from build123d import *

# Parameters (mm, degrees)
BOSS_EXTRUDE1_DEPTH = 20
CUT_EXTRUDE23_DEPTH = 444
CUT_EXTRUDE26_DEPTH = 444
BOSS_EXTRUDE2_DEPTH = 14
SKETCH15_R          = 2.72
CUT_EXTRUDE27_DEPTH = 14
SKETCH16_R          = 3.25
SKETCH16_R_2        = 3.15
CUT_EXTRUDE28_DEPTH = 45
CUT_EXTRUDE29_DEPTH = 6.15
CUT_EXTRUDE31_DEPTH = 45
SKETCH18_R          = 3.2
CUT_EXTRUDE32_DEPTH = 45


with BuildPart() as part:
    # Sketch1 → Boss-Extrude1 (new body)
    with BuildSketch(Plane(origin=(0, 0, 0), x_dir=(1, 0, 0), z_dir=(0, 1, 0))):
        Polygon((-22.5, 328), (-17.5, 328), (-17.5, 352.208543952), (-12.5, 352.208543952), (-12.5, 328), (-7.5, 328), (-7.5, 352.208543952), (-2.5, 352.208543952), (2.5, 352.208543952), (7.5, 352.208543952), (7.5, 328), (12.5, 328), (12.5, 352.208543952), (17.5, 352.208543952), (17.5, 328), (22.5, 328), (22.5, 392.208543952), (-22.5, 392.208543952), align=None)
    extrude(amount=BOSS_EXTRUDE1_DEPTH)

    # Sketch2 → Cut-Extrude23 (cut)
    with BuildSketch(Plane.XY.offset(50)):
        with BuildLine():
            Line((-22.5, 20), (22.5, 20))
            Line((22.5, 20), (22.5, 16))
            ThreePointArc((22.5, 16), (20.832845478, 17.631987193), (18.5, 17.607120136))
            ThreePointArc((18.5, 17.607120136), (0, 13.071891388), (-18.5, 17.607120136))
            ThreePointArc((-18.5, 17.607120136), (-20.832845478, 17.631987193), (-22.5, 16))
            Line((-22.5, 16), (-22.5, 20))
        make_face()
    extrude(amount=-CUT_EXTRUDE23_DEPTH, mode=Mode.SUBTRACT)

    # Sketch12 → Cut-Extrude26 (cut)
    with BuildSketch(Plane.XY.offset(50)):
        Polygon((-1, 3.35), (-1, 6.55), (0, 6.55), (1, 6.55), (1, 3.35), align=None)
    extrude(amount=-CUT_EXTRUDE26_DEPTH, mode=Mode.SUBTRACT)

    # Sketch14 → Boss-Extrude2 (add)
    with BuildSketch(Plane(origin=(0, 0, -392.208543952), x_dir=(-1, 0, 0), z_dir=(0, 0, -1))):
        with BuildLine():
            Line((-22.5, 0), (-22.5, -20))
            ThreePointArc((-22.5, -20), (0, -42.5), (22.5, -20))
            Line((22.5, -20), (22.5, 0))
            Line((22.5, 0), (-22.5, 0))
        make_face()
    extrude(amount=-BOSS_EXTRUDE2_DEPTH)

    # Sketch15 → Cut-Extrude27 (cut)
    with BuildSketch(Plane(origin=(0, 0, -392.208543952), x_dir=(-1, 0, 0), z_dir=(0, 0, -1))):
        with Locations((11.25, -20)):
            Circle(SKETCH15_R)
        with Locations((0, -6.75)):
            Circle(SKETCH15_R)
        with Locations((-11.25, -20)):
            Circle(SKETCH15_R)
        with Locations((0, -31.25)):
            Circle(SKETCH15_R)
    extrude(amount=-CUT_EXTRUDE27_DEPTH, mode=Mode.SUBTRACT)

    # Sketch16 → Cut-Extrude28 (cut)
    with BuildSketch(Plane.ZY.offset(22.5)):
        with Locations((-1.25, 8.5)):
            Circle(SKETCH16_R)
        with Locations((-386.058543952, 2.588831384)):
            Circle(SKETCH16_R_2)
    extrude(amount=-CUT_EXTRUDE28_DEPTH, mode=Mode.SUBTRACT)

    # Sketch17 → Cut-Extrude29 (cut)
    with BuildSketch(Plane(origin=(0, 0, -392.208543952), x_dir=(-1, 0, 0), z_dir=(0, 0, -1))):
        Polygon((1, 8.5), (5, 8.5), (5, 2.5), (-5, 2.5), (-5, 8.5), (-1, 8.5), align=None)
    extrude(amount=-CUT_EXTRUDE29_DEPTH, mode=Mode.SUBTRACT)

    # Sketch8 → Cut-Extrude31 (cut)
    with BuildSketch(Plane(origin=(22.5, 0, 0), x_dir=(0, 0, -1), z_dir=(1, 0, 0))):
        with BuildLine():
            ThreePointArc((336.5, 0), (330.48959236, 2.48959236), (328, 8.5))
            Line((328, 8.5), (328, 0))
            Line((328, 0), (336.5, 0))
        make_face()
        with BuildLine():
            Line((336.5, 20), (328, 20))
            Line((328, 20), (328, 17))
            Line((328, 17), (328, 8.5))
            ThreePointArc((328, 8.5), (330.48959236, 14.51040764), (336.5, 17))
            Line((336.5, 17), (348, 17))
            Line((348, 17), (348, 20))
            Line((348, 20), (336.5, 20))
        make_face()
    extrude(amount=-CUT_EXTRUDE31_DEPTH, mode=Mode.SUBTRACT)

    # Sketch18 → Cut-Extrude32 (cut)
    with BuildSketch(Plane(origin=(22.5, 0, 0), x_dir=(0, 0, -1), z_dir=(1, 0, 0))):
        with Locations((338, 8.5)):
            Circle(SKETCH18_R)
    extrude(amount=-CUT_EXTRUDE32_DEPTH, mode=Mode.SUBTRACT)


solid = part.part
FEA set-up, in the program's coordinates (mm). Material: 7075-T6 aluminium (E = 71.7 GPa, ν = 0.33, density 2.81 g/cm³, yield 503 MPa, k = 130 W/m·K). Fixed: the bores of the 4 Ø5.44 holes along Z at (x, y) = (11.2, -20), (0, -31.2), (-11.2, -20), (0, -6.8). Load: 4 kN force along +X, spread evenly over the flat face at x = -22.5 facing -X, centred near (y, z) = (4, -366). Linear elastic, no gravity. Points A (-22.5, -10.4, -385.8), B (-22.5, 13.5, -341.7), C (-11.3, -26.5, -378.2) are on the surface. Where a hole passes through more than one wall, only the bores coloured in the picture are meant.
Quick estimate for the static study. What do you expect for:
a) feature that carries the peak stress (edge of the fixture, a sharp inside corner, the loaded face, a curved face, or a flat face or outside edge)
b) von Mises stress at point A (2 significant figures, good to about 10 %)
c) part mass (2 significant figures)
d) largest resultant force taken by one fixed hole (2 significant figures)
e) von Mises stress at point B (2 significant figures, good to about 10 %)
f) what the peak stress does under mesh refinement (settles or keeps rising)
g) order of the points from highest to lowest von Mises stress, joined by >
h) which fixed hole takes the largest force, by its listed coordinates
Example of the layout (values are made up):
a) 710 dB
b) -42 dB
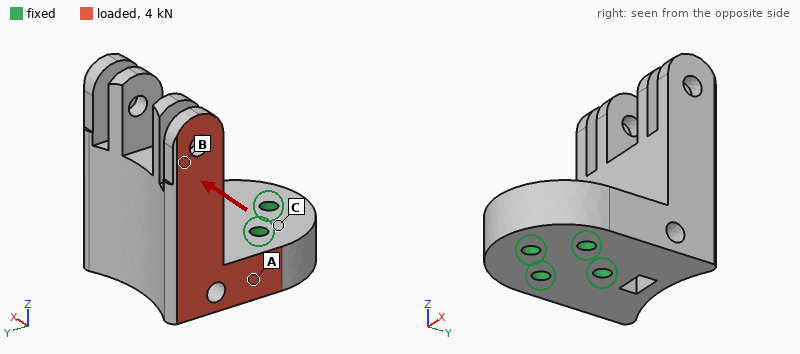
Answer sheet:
a) edge of the fixture
b) 30 MPa
c) 150 g
d) 3.8 kN
e) 70 MPa
f) keeps rising
g) B > A > C
h) (0, -6.8)
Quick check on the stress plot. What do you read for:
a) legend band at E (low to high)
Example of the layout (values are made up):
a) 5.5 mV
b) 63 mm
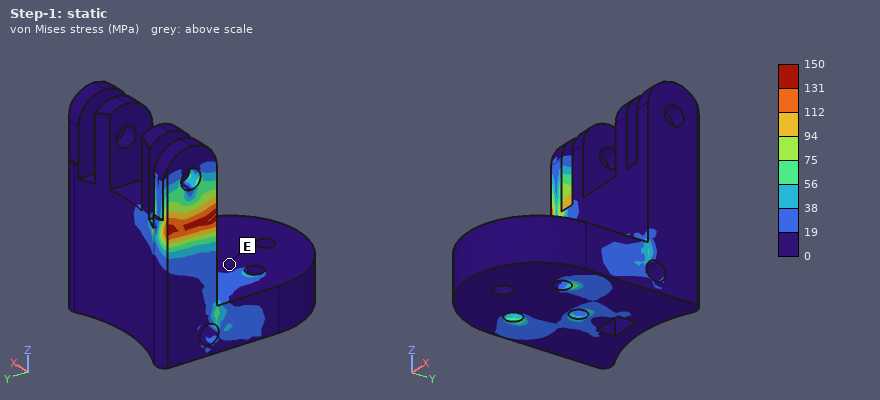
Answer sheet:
a) 0 to 19 MPa
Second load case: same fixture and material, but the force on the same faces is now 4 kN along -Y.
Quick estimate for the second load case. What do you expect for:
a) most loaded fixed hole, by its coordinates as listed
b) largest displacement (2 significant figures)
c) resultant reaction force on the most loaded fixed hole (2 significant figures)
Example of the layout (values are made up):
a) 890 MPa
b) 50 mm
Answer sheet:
a) (-11.2, -20)
b) 0.28 mm
c) 3.5 kN
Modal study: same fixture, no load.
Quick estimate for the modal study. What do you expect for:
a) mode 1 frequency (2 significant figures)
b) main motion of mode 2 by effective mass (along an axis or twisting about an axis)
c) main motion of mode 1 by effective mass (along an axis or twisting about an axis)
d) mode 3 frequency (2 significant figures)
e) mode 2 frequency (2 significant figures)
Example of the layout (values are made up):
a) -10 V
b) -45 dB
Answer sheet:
a) 3100 Hz
b) along X
c) along Y
d) 6300 Hz
e) 4100 Hz
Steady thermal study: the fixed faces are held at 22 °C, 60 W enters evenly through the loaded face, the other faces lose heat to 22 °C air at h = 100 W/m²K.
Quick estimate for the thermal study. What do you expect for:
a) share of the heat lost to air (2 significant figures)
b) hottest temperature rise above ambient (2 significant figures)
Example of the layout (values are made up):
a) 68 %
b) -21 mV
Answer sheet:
a) 22 %
b) 43 K
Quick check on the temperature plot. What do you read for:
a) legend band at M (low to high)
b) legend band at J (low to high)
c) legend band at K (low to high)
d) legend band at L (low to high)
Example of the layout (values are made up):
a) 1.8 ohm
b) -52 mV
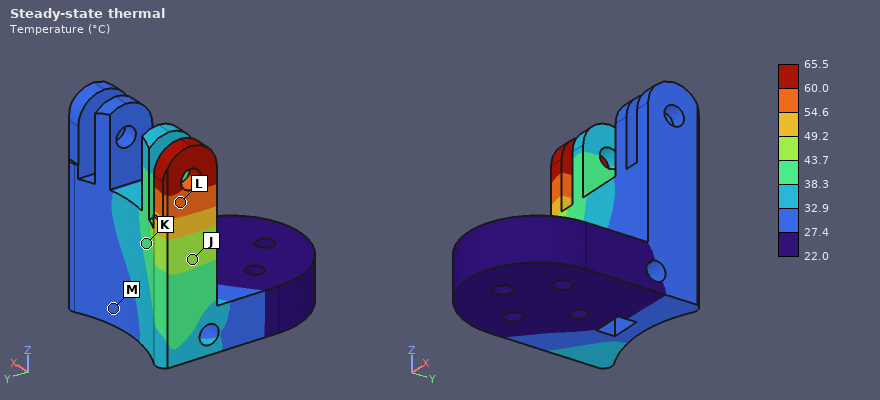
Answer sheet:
a) 27.4 to 32.9 °C
b) 43.7 to 49.2 °C
c) 38.3 to 43.7 °C
d) 54.6 to 60.0 °C
